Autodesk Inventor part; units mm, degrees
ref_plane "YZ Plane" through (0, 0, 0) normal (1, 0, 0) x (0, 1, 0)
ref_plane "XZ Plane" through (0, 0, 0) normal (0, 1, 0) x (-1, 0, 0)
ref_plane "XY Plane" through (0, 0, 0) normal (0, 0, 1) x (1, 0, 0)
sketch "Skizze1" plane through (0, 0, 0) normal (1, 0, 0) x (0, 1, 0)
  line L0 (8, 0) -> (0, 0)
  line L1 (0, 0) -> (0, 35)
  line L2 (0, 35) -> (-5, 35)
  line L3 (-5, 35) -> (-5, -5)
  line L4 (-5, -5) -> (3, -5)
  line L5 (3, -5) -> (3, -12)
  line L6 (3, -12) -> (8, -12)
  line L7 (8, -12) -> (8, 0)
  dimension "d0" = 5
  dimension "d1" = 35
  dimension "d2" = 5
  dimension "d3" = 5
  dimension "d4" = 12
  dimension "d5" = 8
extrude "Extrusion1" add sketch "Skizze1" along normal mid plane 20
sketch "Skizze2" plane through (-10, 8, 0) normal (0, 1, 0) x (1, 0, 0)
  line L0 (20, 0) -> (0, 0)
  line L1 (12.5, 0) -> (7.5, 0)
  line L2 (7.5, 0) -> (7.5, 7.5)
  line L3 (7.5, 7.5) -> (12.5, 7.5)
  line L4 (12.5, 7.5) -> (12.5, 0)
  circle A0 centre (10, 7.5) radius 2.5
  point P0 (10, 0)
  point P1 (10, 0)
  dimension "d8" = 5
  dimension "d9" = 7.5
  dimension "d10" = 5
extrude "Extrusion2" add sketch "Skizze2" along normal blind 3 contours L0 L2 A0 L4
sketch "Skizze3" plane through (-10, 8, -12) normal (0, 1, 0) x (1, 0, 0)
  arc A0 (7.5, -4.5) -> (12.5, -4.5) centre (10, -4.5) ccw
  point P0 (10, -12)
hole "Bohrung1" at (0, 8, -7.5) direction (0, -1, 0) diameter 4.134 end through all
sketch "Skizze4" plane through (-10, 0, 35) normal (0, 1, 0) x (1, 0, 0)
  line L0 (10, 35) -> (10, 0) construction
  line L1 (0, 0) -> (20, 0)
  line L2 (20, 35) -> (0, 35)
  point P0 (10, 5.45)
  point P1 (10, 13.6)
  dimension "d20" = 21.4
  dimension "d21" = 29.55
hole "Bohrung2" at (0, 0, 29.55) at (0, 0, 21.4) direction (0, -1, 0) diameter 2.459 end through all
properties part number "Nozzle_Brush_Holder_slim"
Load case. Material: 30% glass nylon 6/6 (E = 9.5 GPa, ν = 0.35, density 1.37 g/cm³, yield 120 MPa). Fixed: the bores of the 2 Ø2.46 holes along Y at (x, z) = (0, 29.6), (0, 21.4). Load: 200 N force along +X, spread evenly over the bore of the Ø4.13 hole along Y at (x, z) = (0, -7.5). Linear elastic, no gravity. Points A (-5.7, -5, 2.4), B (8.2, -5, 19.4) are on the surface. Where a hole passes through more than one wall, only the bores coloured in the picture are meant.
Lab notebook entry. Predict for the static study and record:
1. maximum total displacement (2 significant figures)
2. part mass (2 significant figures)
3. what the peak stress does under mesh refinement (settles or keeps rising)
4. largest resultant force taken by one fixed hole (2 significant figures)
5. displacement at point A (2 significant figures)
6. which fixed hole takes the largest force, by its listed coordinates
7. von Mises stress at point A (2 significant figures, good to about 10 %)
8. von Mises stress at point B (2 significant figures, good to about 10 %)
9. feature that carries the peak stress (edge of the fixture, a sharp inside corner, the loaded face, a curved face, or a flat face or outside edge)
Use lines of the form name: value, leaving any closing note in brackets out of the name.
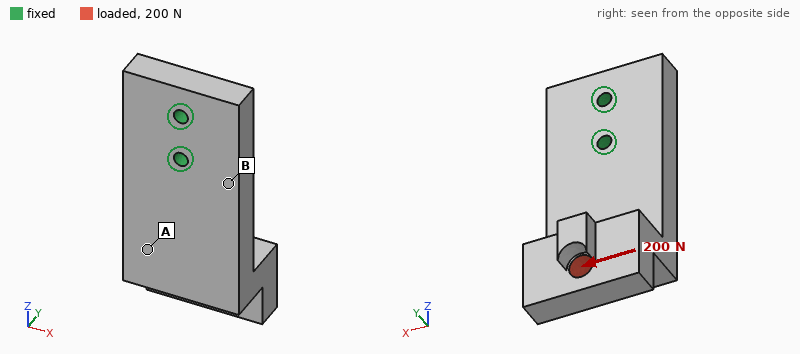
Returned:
maximum total displacement: 0.35 mm
part mass: 7.5 g
what the peak stress does under mesh refinement: keeps rising
largest resultant force taken by one fixed hole: 730 N
displacement at point A: 0.10 mm
which fixed hole takes the largest force, by its listed coordinates: (0, 21.4)
von Mises stress at point A: 8.0 MPa
von Mises stress at point B: 20 MPa
feature that carries the peak stress: edge of the fixture
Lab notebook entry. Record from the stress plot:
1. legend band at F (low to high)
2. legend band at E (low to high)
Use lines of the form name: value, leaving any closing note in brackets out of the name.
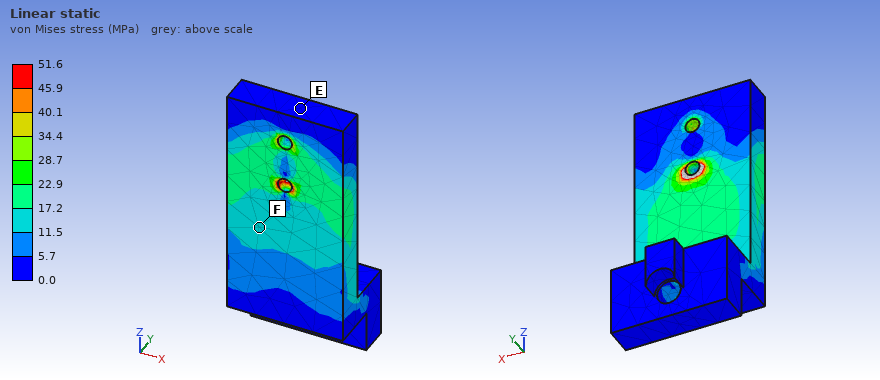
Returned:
legend band at F: 11.5 to 17.2 MPa
legend band at E: 0.0 to 5.7 MPa
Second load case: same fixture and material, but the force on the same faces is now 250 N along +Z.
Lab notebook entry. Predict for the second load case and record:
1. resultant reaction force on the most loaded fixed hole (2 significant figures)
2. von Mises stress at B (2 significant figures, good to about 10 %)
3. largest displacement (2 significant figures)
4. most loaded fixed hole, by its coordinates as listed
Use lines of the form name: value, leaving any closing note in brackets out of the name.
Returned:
resultant reaction force on the most loaded fixed hole: 210 N
von Mises stress at B: 17 MPa
largest displacement: 0.63 mm
most loaded fixed hole, by its coordinates as listed: (0, 21.4)
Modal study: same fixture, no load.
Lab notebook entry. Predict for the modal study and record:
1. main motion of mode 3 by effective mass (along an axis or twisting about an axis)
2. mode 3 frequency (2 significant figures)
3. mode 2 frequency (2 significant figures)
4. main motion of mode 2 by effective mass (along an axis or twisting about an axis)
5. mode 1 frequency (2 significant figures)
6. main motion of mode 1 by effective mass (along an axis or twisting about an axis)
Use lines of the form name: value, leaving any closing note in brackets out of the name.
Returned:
main motion of mode 3 by effective mass: along X
mode 3 frequency: 4700 Hz
mode 2 frequency: 2700 Hz
main motion of mode 2 by effective mass: along X
mode 1 frequency: 1400 Hz
main motion of mode 1 by effective mass: along Y
